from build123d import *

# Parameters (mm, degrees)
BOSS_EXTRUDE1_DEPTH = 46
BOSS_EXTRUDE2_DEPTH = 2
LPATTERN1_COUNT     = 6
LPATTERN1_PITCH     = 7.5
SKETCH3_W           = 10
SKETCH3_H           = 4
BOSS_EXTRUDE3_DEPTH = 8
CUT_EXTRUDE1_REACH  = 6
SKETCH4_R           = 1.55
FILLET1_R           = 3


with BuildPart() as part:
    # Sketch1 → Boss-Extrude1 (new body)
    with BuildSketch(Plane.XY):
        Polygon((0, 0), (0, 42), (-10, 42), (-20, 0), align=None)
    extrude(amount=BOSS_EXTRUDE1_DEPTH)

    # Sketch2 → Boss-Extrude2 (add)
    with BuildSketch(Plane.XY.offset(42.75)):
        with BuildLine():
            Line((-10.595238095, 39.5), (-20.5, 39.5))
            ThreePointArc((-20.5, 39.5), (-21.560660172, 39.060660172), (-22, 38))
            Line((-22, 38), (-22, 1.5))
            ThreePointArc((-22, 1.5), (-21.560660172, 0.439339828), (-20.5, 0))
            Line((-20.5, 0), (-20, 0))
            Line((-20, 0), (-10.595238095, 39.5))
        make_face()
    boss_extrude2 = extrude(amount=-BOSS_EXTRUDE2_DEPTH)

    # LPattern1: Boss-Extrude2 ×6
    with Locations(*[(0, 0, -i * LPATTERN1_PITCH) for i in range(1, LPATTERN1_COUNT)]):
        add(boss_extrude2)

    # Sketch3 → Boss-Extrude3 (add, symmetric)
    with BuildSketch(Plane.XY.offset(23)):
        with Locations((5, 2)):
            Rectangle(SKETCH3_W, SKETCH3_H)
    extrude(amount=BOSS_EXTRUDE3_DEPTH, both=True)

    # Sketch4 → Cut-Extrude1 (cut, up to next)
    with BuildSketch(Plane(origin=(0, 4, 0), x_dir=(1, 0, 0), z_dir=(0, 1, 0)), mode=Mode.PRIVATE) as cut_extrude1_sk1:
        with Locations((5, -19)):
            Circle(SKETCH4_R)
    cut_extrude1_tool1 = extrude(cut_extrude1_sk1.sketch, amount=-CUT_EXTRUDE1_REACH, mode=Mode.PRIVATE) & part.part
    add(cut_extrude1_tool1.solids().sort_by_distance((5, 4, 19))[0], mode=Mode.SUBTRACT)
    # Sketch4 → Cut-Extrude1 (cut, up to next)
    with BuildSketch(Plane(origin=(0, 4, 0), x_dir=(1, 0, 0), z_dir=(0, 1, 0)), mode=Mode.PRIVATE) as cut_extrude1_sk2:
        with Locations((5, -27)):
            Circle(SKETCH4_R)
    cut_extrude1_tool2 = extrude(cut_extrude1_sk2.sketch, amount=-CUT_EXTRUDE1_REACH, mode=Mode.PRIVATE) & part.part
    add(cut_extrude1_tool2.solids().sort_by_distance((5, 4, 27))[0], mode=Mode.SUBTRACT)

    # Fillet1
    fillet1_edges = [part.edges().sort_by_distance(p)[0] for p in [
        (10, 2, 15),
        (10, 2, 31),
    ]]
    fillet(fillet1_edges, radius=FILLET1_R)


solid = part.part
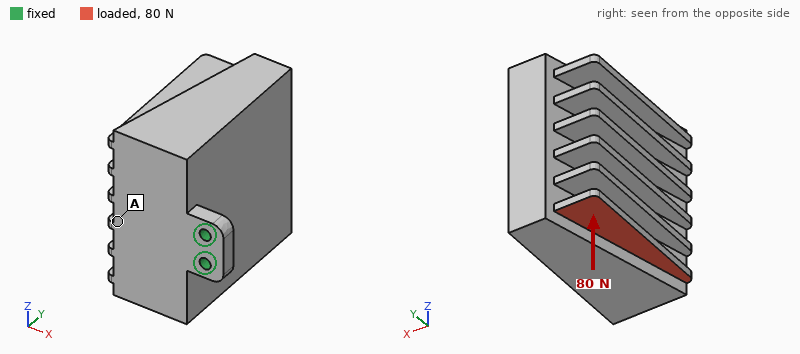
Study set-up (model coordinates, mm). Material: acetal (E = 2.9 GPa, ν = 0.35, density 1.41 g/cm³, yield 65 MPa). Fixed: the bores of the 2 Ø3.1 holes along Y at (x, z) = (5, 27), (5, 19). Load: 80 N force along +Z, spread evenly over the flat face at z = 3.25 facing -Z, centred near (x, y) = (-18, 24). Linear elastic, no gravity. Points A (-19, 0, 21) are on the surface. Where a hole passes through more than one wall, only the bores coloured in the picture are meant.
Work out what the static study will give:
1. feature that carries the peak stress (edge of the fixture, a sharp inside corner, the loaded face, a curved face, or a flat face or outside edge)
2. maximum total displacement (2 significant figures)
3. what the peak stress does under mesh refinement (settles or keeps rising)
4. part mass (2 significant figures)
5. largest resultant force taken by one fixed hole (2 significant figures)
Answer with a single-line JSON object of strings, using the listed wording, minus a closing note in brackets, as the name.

{"feature that carries the peak stress": "edge of the fixture", "maximum total displacement": "0.74 mm", "what the peak stress does under mesh refinement": "keeps rising", "part mass": "46 g", "largest resultant force taken by one fixed hole": "240 N"}
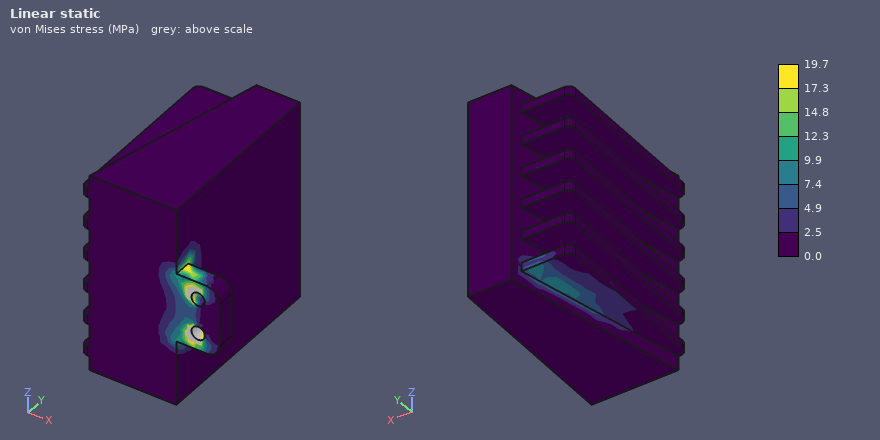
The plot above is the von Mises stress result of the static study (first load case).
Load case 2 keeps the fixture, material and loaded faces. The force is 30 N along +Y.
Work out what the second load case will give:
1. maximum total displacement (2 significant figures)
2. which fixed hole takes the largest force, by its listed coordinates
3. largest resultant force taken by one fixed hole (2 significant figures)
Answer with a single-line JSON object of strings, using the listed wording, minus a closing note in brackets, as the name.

{"maximum total displacement": "0.68 mm", "which fixed hole takes the largest force, by its listed coordinates": "(5, 19)", "largest resultant force taken by one fixed hole": "66 N"}
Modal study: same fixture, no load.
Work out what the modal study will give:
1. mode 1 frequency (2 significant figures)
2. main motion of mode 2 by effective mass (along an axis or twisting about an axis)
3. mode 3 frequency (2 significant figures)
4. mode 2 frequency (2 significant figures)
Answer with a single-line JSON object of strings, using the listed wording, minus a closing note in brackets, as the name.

{"mode 1 frequency": "200 Hz", "main motion of mode 2 by effective mass": "along Z", "mode 3 frequency": "880 Hz", "mode 2 frequency": "360 Hz"}
